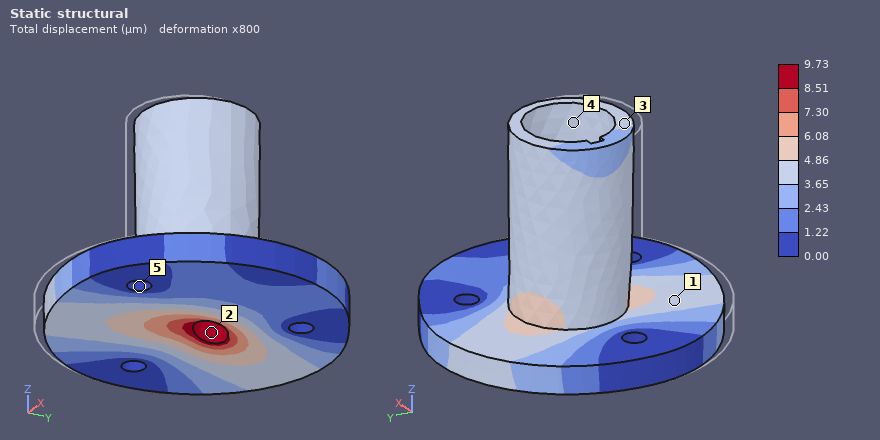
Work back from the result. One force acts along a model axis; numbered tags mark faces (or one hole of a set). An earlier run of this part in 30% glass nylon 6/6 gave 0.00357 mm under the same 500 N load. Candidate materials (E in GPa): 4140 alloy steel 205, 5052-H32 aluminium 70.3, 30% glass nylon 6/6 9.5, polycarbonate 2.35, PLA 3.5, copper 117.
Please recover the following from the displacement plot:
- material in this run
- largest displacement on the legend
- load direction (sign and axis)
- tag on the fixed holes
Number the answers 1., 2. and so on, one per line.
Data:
1. PLA
2. 9.73 µm
3. +Y
4. 5
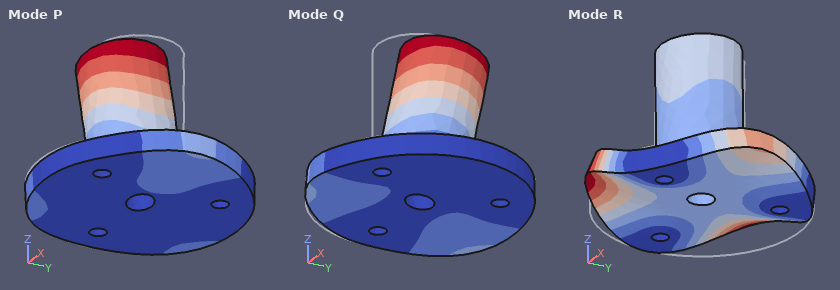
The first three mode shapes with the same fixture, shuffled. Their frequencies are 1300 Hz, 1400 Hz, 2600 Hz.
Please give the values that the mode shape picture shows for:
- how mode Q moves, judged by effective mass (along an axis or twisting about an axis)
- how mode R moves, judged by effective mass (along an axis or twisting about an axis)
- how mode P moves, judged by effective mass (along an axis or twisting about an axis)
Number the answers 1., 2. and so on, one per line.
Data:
1. along Y
2. along Z
3. along X
